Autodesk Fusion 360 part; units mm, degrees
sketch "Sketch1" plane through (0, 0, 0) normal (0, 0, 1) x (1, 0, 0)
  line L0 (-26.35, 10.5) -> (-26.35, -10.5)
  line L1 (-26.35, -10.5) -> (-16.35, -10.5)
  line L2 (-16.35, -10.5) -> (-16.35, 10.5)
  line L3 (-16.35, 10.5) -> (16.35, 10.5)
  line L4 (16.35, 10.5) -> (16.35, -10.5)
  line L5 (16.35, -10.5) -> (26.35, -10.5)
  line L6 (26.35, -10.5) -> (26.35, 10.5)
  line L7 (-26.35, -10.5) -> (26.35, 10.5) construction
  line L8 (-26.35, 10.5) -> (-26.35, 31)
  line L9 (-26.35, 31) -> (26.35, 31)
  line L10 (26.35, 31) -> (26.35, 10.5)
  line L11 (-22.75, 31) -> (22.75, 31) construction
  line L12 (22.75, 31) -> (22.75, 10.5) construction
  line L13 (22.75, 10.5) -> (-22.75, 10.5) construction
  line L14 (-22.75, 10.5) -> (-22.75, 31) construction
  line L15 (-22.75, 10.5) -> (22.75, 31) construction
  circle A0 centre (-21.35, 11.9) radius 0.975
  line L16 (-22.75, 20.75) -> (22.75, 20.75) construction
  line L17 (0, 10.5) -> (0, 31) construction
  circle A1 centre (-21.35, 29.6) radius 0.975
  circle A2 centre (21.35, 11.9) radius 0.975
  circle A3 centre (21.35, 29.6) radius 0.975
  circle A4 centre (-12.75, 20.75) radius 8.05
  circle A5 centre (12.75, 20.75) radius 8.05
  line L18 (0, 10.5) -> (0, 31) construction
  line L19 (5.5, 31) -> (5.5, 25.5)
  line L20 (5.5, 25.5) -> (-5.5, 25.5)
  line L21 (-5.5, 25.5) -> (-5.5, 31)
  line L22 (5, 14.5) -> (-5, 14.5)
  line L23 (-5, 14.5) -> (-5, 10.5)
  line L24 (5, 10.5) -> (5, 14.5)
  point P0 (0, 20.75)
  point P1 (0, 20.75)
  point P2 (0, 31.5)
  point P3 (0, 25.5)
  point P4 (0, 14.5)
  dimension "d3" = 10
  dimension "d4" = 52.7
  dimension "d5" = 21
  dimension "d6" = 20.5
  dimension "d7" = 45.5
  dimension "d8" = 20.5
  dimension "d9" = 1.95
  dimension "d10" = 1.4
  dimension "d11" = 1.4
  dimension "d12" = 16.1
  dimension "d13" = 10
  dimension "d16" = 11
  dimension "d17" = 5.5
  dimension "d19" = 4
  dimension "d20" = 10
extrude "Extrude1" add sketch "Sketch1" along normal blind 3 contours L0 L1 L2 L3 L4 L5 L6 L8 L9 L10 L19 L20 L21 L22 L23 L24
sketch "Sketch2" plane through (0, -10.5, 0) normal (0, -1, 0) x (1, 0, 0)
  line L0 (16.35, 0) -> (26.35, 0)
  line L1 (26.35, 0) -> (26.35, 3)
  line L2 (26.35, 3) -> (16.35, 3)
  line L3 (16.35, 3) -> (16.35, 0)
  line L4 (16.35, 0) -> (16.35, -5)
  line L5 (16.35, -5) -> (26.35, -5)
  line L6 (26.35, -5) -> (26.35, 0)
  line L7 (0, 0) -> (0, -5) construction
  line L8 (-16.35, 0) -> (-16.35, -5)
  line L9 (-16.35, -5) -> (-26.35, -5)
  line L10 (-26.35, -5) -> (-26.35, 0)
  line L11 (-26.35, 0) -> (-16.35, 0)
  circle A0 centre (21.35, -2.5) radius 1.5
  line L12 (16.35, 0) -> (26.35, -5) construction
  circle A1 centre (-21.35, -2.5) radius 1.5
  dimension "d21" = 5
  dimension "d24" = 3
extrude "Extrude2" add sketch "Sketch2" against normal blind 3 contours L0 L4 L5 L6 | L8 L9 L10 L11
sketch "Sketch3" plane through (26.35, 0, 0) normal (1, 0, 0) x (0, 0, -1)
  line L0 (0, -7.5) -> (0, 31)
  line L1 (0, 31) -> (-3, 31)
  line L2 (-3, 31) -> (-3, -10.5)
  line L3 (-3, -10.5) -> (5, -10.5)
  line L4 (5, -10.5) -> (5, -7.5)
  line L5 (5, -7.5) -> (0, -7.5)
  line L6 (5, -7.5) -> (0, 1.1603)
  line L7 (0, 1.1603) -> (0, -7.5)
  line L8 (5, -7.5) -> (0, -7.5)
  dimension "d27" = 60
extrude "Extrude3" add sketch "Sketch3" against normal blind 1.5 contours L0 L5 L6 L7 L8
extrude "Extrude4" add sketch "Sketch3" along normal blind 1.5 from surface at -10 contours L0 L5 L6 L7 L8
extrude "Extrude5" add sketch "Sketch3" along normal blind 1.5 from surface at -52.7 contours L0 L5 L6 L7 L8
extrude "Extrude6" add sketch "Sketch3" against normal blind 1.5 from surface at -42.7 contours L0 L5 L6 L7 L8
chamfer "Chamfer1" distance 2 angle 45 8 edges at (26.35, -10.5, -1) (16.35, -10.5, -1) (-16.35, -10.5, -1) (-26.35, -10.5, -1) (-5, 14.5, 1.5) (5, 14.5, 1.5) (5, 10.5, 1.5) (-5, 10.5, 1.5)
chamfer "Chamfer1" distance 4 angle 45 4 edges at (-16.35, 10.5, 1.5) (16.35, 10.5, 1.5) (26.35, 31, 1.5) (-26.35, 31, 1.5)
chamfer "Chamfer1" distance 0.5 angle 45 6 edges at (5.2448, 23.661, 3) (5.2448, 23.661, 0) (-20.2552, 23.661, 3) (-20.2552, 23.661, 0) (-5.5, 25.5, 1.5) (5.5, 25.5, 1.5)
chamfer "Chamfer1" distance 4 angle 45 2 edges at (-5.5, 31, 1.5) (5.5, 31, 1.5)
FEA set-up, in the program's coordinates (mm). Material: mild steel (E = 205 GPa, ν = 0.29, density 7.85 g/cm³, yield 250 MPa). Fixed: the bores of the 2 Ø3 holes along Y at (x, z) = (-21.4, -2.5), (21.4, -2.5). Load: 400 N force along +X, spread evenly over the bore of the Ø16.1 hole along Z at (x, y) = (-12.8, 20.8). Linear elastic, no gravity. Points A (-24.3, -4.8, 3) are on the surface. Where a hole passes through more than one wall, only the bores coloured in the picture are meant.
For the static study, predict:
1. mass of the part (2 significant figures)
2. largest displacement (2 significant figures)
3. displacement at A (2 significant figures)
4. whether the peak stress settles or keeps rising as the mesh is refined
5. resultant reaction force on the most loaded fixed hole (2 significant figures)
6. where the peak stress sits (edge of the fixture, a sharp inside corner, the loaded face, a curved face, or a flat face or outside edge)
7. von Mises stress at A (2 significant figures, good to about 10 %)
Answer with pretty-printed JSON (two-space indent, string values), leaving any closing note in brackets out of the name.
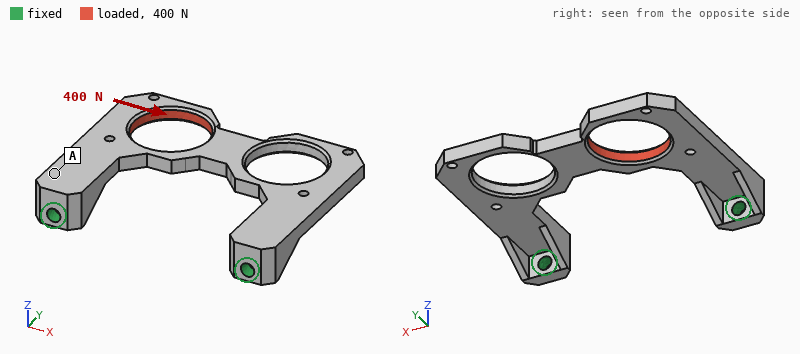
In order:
{
  "mass of the part": "25 g",
  "largest displacement": "34 µm",
  "displacement at A": "5.9 µm",
  "whether the peak stress settles or keeps rising as the mesh is refined": "keeps rising",
  "resultant reaction force on the most loaded fixed hole": "270 N",
  "where the peak stress sits": "edge of the fixture",
  "von Mises stress at A": "21 MPa"
}
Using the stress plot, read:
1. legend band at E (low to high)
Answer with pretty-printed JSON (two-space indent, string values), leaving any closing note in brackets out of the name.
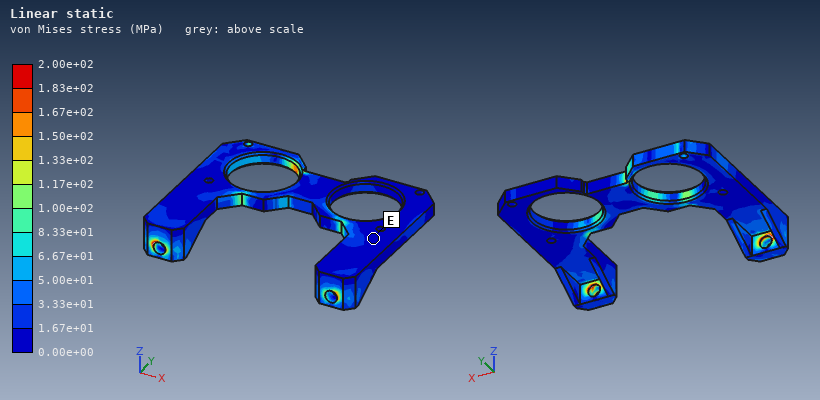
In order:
{
  "legend band at E": "0.00e+00 to 1.67e+01 MPa"
}
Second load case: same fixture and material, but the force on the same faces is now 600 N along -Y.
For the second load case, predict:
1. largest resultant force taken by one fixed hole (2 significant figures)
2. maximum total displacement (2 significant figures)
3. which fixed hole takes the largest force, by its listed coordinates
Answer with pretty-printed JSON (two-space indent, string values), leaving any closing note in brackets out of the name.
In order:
{
  "largest resultant force taken by one fixed hole": "490 N",
  "maximum total displacement": "24 µm",
  "which fixed hole takes the largest force, by its listed coordinates": "(-21.4, -2.5)"
}
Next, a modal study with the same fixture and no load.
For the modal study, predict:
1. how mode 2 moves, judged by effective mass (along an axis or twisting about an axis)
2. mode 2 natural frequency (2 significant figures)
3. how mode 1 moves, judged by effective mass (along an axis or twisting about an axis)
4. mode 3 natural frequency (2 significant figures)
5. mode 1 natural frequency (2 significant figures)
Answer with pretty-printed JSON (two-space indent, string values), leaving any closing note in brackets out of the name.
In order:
{
  "how mode 2 moves, judged by effective mass": "twisting about Y",
  "mode 2 natural frequency": "2800 Hz",
  "how mode 1 moves, judged by effective mass": "along Z",
  "mode 3 natural frequency": "5300 Hz",
  "mode 1 natural frequency": "1600 Hz"
}
